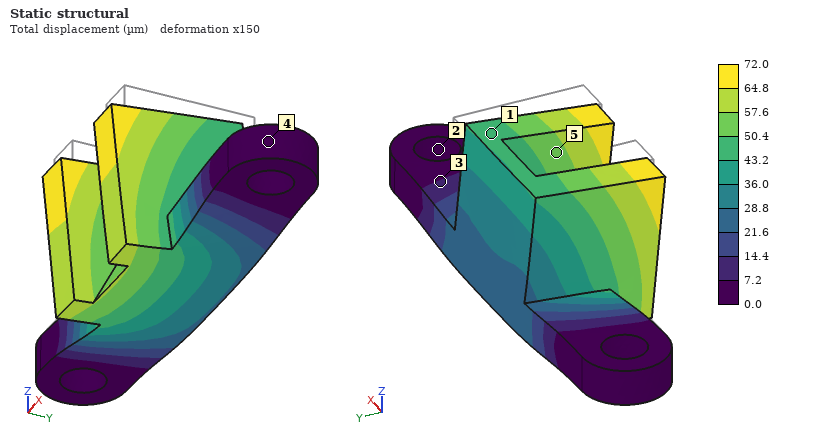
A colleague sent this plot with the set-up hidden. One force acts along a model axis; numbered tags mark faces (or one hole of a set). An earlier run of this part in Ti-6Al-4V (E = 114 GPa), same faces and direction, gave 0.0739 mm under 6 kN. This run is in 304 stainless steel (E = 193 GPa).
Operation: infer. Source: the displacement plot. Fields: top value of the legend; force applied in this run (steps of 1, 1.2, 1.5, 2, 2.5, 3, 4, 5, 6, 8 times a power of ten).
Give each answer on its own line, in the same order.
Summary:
72.0 µm
10 kN
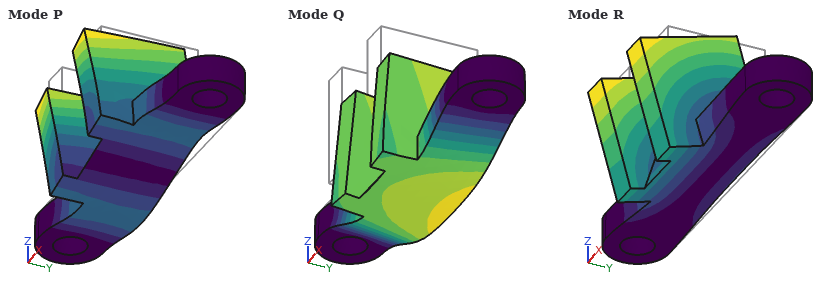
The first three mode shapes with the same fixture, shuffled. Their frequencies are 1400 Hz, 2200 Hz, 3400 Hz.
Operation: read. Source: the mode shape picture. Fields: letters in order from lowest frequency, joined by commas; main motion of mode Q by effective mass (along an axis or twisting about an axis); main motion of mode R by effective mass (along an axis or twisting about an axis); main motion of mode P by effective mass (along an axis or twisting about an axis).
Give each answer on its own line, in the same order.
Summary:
R, Q, P
along Z
along Y
along X
